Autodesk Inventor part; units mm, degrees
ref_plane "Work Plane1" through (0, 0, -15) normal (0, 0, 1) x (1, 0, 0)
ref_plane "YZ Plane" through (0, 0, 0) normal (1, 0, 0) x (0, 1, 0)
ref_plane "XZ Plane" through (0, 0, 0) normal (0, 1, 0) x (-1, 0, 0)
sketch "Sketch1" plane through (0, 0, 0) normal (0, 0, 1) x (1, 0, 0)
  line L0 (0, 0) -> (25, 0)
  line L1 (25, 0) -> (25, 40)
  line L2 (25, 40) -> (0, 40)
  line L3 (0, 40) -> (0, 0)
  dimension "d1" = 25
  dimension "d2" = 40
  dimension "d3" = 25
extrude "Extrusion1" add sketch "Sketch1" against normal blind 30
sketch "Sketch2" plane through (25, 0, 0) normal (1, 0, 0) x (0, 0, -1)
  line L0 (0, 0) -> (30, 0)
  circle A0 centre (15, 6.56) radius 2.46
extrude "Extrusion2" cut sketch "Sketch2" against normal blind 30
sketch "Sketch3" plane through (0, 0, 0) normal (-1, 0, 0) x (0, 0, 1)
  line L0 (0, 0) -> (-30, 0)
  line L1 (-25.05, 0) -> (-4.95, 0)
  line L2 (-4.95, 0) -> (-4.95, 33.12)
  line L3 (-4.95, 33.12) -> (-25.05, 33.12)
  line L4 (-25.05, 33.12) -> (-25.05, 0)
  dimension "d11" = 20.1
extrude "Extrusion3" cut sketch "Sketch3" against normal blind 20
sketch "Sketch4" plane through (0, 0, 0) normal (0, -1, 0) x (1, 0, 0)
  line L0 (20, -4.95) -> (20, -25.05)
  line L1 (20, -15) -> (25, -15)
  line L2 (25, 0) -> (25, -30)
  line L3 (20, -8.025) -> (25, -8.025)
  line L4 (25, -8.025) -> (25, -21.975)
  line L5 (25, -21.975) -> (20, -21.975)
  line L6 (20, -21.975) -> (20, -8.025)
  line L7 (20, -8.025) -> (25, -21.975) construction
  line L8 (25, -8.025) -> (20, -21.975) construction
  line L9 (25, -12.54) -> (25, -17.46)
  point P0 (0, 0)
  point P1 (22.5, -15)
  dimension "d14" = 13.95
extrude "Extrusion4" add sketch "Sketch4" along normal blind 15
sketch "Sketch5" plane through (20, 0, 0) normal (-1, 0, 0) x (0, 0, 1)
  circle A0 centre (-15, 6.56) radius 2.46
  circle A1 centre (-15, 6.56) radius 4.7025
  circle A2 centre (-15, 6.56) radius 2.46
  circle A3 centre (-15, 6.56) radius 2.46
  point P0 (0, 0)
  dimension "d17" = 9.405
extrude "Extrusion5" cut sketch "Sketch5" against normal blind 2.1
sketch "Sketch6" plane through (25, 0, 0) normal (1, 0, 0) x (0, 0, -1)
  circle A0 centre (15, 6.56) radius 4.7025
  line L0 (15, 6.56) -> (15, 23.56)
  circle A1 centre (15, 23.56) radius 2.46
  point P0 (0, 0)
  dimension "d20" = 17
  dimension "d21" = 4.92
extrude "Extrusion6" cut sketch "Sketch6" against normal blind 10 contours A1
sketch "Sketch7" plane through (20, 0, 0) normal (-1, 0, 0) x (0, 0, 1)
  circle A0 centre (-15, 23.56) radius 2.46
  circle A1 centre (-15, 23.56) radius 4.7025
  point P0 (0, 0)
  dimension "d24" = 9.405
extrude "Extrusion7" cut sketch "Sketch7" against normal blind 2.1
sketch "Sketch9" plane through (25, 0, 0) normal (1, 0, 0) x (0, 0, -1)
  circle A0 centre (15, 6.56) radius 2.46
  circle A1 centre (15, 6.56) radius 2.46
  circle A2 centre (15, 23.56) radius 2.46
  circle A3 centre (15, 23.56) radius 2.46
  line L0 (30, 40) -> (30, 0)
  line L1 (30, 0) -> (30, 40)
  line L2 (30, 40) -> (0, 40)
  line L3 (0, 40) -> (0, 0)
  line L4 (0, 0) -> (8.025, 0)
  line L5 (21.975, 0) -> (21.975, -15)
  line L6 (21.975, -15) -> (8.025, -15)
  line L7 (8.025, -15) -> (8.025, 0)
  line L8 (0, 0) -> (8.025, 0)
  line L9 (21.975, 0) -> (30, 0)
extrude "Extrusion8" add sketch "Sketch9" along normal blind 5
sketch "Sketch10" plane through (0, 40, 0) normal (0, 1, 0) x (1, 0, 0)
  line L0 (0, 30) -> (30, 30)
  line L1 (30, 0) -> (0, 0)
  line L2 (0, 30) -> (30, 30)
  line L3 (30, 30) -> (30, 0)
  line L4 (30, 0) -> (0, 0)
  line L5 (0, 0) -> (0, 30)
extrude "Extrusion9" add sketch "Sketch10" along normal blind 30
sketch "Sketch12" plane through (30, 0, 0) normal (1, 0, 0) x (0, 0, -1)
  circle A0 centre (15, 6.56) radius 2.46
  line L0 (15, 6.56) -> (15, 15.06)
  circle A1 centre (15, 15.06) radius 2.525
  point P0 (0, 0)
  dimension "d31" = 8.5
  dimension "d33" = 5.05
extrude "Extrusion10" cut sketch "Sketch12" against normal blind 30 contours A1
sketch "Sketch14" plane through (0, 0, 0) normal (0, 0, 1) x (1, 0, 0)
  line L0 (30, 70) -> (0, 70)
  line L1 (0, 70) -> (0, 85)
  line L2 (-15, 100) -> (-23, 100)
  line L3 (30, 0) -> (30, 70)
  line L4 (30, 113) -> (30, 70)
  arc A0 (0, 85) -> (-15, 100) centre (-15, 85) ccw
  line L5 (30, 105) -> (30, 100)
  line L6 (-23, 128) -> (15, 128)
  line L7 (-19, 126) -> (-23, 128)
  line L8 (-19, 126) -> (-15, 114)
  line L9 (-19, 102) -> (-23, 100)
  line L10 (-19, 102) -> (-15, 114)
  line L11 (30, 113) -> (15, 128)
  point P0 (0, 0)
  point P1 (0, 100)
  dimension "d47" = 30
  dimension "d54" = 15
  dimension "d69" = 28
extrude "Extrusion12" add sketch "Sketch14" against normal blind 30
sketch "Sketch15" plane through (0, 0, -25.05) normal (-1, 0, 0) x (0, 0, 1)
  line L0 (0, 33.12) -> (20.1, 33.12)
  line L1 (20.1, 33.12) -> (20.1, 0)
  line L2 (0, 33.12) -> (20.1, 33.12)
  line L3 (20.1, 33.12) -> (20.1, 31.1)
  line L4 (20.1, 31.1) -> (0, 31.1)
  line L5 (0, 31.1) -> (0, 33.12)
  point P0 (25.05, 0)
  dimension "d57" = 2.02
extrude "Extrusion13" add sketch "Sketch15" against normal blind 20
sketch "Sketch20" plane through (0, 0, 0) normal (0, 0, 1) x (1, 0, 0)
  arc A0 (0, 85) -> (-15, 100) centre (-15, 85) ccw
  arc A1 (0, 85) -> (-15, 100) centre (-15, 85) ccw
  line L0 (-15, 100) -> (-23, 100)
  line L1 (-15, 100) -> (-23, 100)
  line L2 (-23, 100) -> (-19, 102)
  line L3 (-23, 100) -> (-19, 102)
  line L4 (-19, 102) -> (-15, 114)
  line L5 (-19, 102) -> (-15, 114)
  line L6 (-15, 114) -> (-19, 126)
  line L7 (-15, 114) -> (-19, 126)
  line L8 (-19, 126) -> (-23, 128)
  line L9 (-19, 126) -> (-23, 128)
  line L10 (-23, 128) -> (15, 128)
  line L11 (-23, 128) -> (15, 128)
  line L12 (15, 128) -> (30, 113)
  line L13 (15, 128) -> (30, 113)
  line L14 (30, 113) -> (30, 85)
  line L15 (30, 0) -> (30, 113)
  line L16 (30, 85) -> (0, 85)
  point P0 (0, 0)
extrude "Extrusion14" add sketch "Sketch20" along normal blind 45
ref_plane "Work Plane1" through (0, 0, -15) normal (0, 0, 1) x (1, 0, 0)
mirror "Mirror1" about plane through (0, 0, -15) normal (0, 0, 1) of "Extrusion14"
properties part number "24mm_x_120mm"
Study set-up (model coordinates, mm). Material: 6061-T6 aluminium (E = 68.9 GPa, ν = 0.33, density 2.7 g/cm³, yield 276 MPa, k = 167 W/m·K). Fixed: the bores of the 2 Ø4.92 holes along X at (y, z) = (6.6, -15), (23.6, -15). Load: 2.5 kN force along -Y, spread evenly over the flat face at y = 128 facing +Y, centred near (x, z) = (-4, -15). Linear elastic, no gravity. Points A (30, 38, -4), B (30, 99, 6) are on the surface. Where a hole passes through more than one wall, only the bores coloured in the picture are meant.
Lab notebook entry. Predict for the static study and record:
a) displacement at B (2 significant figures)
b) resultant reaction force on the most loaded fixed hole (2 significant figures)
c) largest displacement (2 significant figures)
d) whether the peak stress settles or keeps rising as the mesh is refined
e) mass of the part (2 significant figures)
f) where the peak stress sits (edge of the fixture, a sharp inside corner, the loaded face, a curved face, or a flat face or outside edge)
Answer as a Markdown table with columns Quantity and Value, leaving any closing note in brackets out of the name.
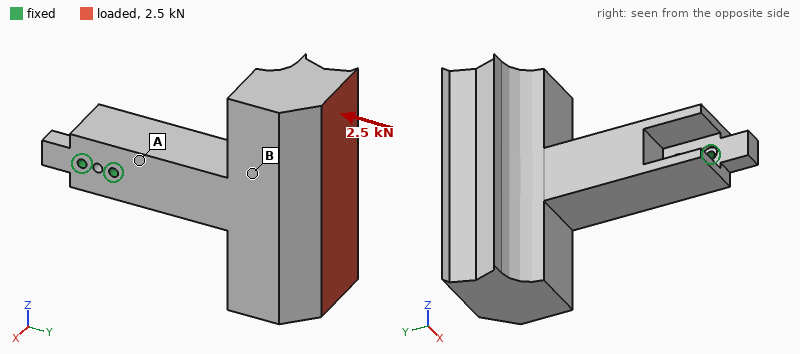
| Quantity | Value |
|---|---|
| displacement at B | 0.14 mm |
| resultant reaction force on the most loaded fixed hole | 3.4 kN |
| largest displacement | 0.24 mm |
| whether the peak stress settles or keeps rising as the mesh is refined | keeps rising |
| mass of the part | 730 g |
| where the peak stress sits | edge of the fixture |
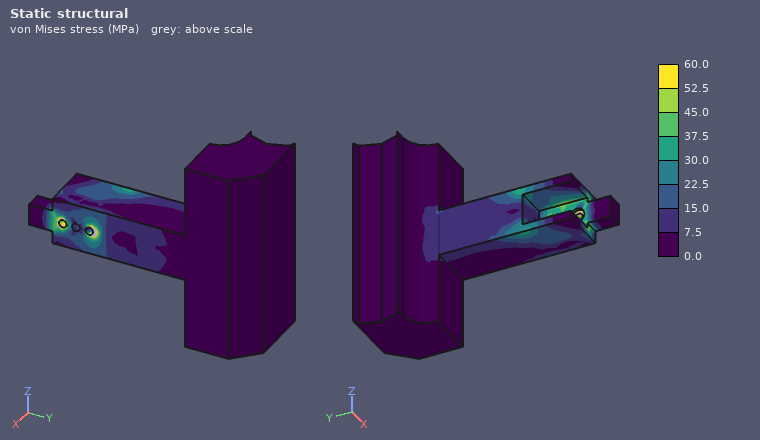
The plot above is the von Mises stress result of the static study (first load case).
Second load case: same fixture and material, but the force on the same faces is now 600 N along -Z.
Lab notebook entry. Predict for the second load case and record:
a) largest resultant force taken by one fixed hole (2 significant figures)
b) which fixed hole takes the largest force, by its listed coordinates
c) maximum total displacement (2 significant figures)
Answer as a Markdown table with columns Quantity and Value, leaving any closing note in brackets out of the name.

| Quantity | Value |
|---|---|
| largest resultant force taken by one fixed hole | 3.3 kN |
| which fixed hole takes the largest force, by its listed coordinates | (23.6, -15) |
| maximum total displacement | 0.19 mm |
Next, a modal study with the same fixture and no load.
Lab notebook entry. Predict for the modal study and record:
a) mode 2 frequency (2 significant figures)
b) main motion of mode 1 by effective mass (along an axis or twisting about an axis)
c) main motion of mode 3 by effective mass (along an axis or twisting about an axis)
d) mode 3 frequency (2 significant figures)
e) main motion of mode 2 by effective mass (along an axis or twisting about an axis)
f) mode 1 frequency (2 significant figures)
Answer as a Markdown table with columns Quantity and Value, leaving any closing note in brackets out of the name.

| Quantity | Value |
|---|---|
| mode 2 frequency | 490 Hz |
| main motion of mode 1 by effective mass | along X |
| main motion of mode 3 by effective mass | twisting about Y |
| mode 3 frequency | 700 Hz |
| main motion of mode 2 by effective mass | along Z |
| mode 1 frequency | 460 Hz |
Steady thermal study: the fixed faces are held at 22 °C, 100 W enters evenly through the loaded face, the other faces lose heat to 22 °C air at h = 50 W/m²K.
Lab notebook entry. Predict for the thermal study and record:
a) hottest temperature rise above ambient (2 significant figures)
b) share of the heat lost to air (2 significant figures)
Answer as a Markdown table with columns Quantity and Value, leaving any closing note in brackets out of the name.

| Quantity | Value |
|---|---|
| hottest temperature rise above ambient | 44 K |
| share of the heat lost to air | 48 % |
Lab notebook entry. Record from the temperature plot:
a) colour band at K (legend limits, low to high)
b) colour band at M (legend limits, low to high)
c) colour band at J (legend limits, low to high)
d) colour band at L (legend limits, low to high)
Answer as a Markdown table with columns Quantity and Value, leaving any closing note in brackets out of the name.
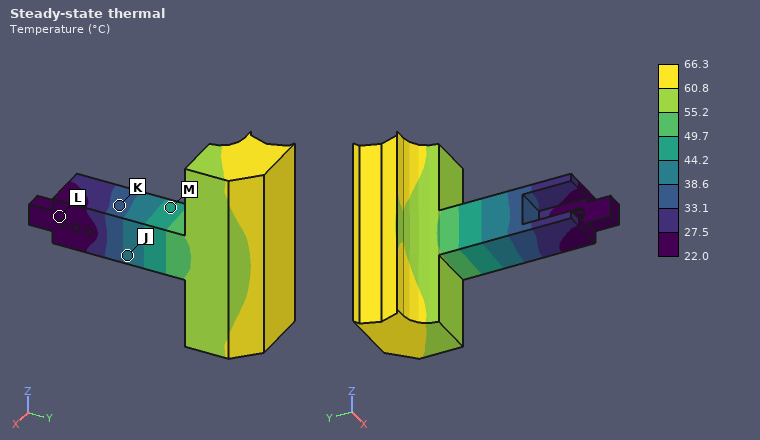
| Quantity | Value |
|---|---|
| colour band at K | 33.1 to 38.6 °C |
| colour band at M | 44.2 to 49.7 °C |
| colour band at J | 38.6 to 44.2 °C |
| colour band at L | 22.0 to 27.5 °C |
